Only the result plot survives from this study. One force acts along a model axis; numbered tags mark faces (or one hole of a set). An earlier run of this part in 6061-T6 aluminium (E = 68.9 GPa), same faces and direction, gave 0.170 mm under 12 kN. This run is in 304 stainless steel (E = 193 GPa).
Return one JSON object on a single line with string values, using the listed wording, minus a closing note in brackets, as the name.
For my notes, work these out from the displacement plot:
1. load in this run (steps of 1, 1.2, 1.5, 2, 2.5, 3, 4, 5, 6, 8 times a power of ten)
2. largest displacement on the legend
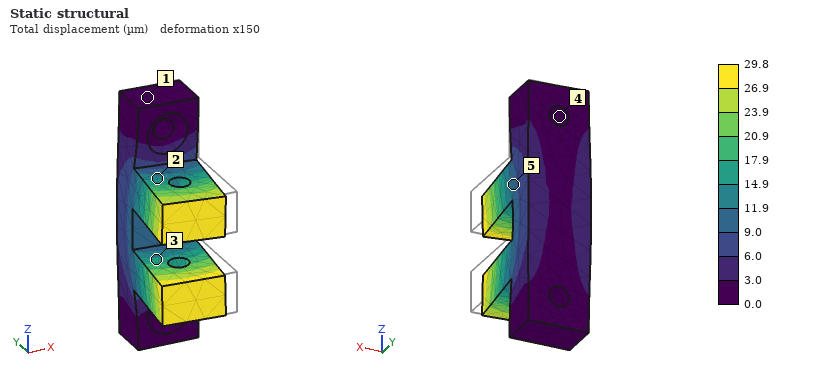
{"load in this run": "6 kN", "largest displacement on the legend": "29.8 µm"}
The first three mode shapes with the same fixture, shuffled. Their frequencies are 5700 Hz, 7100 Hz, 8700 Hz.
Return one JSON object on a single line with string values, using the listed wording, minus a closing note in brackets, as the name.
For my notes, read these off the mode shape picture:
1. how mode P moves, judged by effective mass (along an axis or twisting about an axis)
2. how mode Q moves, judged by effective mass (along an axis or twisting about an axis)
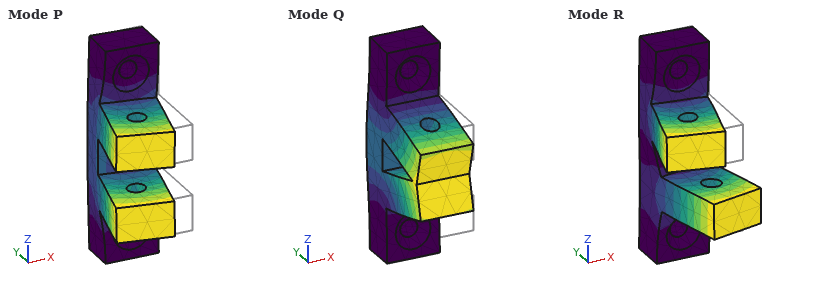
{"how mode P moves, judged by effective mass": "along X", "how mode Q moves, judged by effective mass": "along Y"}
